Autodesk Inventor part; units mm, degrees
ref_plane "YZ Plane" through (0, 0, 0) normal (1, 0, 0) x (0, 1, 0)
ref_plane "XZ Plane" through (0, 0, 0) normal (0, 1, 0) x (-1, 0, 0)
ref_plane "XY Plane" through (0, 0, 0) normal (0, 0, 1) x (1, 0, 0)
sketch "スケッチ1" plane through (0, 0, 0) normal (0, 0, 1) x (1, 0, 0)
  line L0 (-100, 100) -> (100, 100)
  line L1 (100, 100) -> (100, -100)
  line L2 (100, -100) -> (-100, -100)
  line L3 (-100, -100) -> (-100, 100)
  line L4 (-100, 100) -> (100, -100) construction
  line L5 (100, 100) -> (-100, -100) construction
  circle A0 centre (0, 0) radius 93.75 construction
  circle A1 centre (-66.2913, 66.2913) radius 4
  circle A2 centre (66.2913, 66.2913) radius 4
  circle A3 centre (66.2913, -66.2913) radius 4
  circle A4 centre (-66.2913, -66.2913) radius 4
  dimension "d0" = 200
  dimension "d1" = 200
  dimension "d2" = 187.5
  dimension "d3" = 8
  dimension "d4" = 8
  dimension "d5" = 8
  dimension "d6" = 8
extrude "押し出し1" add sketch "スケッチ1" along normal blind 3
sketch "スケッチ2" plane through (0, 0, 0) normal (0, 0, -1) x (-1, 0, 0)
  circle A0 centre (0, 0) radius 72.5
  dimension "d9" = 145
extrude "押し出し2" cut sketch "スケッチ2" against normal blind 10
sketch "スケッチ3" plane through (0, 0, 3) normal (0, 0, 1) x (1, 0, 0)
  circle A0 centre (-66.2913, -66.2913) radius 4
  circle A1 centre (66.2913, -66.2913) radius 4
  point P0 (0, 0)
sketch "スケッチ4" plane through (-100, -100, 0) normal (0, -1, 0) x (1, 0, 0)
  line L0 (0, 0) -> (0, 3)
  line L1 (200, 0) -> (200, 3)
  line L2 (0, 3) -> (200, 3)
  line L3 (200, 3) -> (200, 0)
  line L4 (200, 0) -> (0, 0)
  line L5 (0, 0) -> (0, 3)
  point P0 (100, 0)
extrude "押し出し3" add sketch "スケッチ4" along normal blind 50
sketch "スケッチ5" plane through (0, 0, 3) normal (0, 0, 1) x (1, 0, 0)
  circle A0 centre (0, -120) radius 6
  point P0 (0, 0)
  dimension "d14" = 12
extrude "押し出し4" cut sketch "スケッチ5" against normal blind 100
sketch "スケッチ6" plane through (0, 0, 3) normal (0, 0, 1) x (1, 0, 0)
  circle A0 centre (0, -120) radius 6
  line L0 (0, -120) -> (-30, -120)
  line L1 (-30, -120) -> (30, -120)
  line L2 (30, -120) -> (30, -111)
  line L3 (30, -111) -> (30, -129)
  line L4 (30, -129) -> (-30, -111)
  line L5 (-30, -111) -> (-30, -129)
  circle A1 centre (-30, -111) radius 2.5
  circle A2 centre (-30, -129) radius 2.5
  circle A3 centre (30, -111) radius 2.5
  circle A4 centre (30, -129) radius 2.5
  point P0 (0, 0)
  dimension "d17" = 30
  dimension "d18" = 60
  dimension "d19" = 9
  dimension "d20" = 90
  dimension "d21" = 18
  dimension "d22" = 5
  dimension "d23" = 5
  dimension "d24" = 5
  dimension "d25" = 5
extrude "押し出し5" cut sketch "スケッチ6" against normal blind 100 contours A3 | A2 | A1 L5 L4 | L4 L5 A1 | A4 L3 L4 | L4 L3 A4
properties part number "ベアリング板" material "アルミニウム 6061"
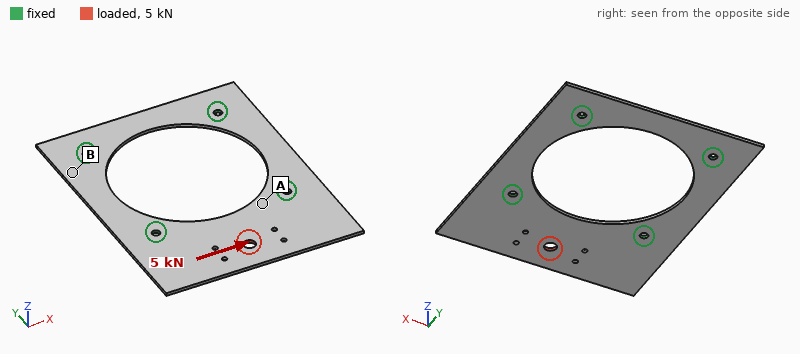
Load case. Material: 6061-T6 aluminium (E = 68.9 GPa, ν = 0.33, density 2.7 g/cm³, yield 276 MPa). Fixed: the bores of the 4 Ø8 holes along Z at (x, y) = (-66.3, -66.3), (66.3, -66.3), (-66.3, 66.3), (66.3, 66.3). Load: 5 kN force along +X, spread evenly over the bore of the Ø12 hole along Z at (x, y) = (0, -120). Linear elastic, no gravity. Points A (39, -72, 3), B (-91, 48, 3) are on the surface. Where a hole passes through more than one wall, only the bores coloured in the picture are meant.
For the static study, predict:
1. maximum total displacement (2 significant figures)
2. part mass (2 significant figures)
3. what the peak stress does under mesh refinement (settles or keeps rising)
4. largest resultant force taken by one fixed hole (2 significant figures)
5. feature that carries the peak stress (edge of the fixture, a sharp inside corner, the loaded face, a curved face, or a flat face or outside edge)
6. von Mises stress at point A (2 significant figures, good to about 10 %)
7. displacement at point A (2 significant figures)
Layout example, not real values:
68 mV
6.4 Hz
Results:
46 µm
270 g
keeps rising
3.0 kN
edge of the fixture
22 MPa
11 µm
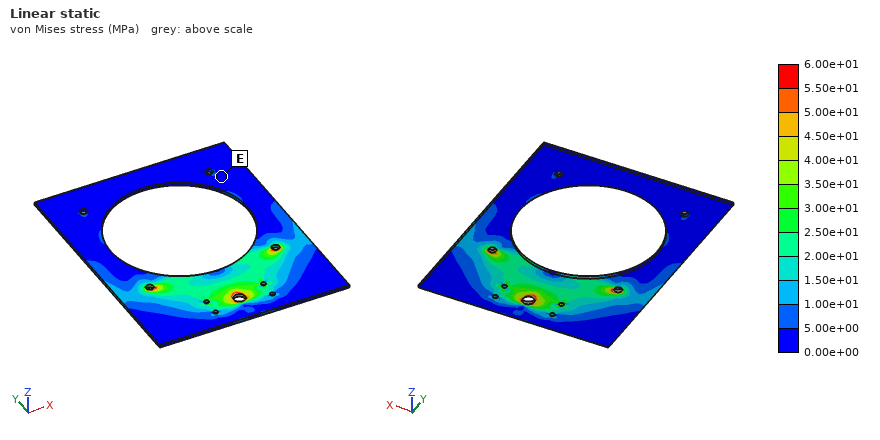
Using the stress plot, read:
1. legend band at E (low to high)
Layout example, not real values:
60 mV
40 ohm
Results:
0.00e+00 to 5.00e+00 MPa
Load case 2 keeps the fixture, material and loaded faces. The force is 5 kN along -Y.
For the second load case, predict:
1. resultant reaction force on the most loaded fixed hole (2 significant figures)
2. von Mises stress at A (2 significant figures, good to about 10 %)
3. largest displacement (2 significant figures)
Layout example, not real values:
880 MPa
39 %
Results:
3.0 kN
20 MPa
50 µm
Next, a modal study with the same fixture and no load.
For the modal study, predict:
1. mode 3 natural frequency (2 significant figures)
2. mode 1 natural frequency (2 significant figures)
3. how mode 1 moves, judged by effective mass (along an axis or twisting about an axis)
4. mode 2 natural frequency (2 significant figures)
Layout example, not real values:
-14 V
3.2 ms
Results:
680 Hz
290 Hz
along Z
470 Hz
